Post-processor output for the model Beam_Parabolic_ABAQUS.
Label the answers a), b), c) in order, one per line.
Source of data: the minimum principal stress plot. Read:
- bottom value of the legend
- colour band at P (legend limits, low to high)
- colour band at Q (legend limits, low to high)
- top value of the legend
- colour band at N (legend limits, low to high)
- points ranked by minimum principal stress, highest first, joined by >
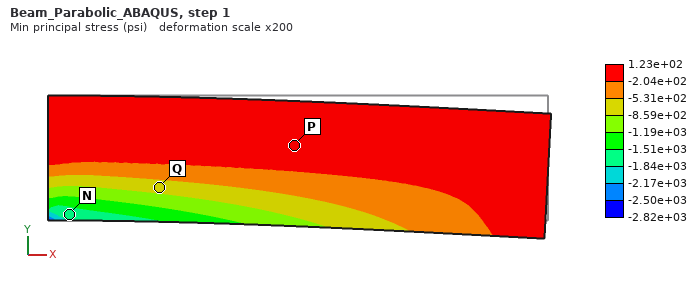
a) -2.82e+03 psi
b) -2.04e+02 to 1.23e+02 psi
c) -8.59e+02 to -5.31e+02 psi
d) 1.23e+02 psi
e) -1.84e+03 to -1.51e+03 psi
f) P > Q > N
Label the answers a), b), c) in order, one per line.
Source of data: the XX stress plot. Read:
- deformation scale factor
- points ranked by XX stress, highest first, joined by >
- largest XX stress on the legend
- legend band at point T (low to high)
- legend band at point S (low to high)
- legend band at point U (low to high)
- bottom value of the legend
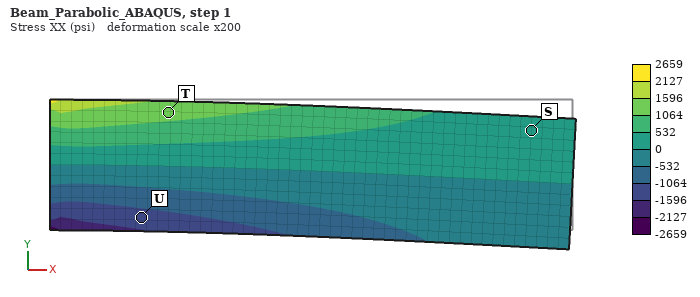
a) 200
b) T > S > U
c) 2659 psi
d) 1064 to 1596 psi
e) 0 to 532 psi
f) -1596 to -1064 psi
g) -2659 psi
